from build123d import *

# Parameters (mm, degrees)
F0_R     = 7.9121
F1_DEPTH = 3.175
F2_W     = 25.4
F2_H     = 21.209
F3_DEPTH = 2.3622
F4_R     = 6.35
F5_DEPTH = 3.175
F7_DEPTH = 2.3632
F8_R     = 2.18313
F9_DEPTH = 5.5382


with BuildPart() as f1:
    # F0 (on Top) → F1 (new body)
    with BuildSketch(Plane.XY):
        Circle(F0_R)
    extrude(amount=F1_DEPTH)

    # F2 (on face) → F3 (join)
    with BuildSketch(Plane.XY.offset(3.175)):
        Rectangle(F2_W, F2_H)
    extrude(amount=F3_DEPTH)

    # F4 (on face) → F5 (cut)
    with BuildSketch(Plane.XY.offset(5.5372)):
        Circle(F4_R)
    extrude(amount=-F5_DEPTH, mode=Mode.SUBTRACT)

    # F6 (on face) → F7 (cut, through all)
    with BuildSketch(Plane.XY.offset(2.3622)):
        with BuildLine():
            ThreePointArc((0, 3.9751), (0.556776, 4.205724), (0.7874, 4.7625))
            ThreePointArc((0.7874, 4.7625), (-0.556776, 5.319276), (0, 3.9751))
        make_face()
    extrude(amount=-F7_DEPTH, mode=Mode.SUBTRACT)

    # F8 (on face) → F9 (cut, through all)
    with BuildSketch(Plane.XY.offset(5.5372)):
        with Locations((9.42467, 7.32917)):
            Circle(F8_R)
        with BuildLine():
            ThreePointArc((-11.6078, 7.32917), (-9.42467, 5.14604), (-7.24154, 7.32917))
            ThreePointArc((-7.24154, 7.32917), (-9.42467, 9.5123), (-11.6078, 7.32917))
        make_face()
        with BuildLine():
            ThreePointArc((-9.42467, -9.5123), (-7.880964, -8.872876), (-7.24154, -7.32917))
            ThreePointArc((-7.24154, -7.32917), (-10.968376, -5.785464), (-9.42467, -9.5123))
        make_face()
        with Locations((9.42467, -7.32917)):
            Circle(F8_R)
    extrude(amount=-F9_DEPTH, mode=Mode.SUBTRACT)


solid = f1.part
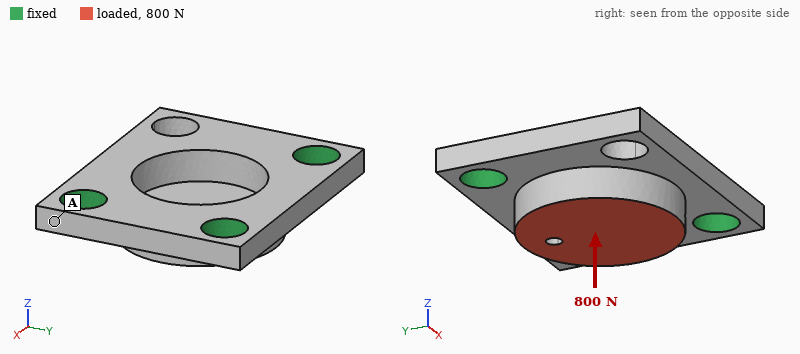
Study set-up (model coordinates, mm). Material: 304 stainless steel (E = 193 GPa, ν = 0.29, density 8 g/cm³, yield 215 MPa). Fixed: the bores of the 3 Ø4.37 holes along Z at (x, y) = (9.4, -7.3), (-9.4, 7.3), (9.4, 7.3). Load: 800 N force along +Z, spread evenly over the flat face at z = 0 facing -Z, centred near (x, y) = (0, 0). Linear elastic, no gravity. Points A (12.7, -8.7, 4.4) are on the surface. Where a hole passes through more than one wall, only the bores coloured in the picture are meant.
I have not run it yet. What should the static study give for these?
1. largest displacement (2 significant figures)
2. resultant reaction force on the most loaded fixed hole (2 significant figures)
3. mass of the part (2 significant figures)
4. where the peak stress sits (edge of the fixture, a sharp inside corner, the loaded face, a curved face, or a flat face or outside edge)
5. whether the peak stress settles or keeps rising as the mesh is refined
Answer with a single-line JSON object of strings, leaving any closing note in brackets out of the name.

{"largest displacement": "11 µm", "resultant reaction force on the most loaded fixed hole": "470 N", "mass of the part": "11 g", "where the peak stress sits": "edge of the fixture", "whether the peak stress settles or keeps rising as the mesh is refined": "keeps rising"}
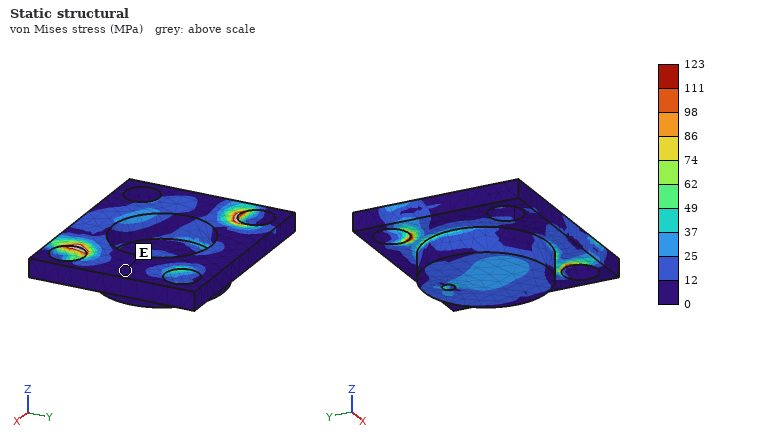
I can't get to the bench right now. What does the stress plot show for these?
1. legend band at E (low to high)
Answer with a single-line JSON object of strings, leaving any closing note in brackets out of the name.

{"legend band at E": "0 to 12 MPa"}
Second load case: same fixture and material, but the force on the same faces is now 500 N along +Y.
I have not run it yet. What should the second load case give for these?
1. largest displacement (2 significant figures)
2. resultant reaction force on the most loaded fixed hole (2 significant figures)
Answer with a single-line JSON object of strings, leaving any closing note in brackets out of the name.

{"largest displacement": "5.2 µm", "resultant reaction force on the most loaded fixed hole": "250 N"}
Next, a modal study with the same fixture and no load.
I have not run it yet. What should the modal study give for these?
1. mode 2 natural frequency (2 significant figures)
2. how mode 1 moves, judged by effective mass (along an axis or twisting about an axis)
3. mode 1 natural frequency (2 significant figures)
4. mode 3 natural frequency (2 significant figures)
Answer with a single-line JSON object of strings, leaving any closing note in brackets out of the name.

{"mode 2 natural frequency": "34 kHz", "how mode 1 moves, judged by effective mass": "along Z", "mode 1 natural frequency": "16 kHz", "mode 3 natural frequency": "43 kHz"}
